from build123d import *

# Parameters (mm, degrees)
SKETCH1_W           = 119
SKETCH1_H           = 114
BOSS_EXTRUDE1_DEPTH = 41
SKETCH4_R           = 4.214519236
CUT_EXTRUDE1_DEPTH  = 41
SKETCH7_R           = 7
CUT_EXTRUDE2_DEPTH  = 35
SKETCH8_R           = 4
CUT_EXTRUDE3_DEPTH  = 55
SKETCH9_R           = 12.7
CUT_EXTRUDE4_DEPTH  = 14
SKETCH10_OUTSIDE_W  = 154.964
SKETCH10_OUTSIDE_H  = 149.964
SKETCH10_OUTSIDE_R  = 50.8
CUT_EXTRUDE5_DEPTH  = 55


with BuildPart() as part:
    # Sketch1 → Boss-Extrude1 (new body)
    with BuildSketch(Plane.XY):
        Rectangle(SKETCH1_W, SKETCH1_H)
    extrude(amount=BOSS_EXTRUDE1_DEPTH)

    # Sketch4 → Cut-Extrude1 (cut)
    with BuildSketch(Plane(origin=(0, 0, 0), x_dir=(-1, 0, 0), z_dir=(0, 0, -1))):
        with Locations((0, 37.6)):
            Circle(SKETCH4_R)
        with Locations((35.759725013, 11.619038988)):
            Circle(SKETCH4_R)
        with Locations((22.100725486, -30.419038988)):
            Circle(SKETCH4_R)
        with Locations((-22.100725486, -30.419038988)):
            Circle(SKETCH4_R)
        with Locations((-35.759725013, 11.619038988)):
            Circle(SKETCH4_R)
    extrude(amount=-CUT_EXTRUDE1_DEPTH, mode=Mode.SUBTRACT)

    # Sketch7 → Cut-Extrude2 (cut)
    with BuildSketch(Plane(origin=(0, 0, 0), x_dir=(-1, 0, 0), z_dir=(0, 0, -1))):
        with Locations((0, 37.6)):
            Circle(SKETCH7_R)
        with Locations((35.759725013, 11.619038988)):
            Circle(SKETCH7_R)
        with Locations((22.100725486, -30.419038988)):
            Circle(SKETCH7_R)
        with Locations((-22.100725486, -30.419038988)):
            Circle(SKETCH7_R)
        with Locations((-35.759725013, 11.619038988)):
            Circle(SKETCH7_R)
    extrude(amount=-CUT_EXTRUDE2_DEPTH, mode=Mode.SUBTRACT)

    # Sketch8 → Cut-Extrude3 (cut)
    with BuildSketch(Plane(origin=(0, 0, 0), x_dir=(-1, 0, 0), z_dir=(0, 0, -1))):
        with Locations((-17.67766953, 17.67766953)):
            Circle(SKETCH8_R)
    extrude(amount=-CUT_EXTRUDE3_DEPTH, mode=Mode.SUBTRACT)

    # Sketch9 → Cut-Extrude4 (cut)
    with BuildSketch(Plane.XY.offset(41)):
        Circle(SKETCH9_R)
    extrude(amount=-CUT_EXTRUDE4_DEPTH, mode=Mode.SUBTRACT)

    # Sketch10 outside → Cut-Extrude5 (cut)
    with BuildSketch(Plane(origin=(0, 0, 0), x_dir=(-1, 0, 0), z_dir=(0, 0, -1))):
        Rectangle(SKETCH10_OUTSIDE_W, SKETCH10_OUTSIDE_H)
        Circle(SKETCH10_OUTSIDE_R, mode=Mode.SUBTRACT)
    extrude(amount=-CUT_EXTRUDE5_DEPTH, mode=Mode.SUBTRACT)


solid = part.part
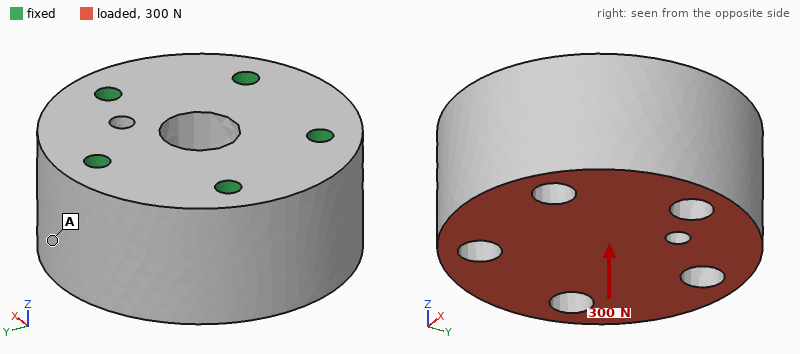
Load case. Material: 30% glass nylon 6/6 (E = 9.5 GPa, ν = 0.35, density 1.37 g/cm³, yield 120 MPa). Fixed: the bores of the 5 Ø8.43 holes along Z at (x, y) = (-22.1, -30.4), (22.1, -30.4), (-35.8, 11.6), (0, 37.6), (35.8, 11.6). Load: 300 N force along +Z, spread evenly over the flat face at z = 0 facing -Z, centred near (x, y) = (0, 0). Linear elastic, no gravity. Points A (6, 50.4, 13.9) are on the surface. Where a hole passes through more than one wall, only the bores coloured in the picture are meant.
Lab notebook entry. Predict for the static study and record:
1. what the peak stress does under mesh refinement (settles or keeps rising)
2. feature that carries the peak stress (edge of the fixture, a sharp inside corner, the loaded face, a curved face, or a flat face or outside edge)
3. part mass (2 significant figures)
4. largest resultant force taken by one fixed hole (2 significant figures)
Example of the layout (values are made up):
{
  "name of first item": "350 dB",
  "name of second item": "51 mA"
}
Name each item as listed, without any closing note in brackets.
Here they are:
{
  "what the peak stress does under mesh refinement": "keeps rising",
  "feature that carries the peak stress": "edge of the fixture",
  "part mass": "400 g",
  "largest resultant force taken by one fixed hole": "61 N"
}
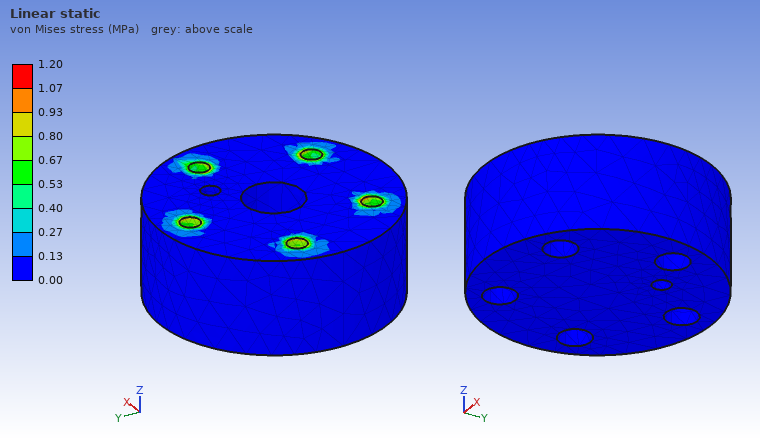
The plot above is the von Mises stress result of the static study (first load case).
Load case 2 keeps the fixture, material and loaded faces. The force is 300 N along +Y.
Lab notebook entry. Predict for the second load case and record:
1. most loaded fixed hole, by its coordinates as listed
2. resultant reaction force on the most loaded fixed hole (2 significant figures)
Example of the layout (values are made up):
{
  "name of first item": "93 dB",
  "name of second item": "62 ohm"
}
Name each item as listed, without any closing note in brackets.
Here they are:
{
  "most loaded fixed hole, by its coordinates as listed": "(0, 37.6)",
  "resultant reaction force on the most loaded fixed hole": "130 N"
}
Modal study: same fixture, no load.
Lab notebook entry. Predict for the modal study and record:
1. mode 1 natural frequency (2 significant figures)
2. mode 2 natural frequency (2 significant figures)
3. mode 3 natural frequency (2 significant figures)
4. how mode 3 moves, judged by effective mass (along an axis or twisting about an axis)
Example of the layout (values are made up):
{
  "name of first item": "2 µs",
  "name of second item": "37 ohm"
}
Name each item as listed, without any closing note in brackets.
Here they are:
{
  "mode 1 natural frequency": "4000 Hz",
  "mode 2 natural frequency": "4000 Hz",
  "mode 3 natural frequency": "5400 Hz",
  "how mode 3 moves, judged by effective mass": "along Z"
}
